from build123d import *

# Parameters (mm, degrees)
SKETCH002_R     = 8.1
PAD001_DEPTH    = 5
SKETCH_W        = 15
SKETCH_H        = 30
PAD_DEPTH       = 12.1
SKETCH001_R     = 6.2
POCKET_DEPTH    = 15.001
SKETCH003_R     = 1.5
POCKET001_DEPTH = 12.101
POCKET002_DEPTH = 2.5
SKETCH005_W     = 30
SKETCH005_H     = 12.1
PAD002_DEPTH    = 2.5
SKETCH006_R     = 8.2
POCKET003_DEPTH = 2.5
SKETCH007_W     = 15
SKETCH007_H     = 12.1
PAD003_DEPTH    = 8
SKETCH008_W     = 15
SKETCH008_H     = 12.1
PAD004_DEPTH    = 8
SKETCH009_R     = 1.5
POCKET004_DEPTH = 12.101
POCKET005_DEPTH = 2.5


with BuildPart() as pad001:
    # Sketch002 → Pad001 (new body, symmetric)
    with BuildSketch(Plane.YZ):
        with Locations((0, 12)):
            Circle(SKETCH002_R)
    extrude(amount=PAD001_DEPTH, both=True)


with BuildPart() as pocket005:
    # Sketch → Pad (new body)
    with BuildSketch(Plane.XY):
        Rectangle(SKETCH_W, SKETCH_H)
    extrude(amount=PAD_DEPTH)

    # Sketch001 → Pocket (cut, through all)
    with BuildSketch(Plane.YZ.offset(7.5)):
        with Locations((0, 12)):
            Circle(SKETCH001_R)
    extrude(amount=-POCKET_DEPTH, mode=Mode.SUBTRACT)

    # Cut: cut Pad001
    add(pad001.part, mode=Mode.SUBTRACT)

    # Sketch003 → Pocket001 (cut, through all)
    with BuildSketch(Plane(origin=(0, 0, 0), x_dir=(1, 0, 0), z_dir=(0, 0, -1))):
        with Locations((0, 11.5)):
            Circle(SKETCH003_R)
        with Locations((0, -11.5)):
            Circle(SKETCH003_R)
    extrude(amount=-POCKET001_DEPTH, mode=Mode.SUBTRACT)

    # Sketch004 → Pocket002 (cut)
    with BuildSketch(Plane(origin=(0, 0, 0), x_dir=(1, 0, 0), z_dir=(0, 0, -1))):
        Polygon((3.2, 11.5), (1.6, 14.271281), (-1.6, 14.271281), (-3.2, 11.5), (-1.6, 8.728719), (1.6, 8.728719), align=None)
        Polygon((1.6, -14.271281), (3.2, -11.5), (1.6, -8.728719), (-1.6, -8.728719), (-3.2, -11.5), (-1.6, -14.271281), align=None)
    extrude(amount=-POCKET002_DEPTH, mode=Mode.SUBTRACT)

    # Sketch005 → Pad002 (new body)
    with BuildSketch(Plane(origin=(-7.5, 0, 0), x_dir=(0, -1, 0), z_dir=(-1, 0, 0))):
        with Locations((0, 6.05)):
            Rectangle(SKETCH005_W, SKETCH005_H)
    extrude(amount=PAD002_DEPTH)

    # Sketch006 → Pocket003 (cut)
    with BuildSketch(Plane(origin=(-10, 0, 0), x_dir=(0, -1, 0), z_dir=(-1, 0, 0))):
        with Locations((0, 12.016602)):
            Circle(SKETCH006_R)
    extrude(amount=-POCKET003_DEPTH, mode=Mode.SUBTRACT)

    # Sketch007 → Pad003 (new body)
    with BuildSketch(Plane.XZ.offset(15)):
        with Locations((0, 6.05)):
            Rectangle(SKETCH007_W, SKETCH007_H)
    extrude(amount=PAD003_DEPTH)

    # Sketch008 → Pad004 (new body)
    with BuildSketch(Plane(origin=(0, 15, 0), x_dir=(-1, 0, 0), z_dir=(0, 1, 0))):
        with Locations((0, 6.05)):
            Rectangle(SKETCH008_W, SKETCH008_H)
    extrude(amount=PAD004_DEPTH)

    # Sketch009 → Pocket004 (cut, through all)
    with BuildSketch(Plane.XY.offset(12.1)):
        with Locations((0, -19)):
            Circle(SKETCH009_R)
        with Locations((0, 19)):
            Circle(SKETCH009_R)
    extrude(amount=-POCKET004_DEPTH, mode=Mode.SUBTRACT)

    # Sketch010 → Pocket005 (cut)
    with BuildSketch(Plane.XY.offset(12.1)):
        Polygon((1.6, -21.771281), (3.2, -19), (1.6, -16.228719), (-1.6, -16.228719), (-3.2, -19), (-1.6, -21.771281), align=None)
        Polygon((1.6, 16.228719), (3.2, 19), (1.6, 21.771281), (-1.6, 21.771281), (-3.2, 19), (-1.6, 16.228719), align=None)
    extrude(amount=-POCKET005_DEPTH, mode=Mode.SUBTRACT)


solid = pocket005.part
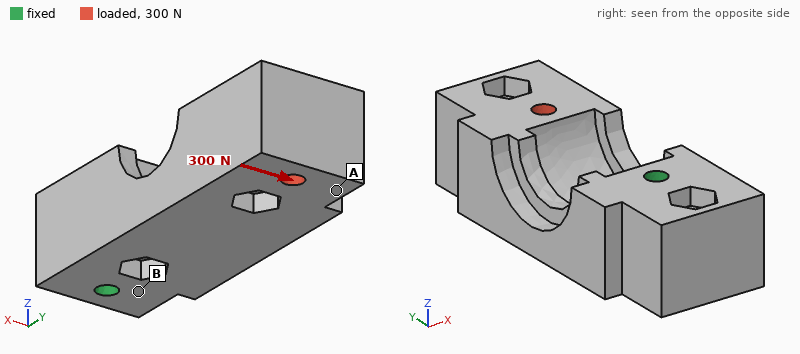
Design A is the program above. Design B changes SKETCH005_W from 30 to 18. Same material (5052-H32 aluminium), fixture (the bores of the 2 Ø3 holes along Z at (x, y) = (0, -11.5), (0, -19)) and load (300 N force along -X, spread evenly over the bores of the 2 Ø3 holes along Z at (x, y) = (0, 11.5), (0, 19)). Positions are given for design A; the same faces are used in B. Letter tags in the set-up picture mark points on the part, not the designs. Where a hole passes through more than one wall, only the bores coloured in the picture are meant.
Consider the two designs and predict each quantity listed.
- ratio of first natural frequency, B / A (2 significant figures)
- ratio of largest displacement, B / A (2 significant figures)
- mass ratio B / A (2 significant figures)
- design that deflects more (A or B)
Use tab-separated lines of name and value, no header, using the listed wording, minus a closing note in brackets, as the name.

ratio of first natural frequency, B / A	1.0
ratio of largest displacement, B / A	1.1
mass ratio B / A	0.95
design that deflects more	B
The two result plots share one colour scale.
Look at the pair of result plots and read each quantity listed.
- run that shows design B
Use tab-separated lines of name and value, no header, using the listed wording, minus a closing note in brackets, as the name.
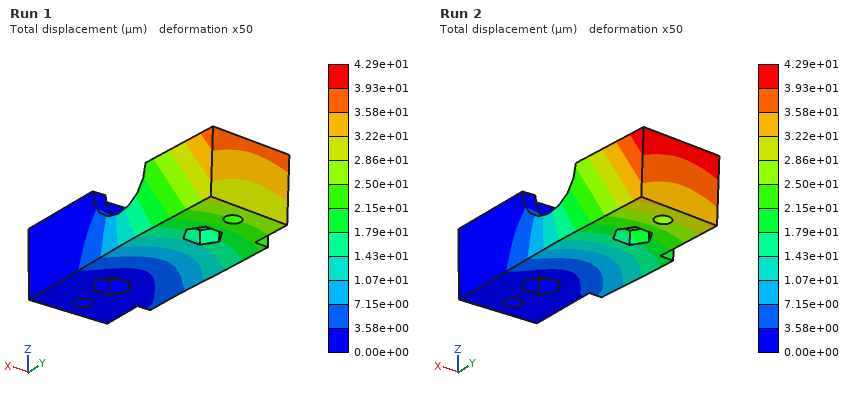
run that shows design B	Run 2
